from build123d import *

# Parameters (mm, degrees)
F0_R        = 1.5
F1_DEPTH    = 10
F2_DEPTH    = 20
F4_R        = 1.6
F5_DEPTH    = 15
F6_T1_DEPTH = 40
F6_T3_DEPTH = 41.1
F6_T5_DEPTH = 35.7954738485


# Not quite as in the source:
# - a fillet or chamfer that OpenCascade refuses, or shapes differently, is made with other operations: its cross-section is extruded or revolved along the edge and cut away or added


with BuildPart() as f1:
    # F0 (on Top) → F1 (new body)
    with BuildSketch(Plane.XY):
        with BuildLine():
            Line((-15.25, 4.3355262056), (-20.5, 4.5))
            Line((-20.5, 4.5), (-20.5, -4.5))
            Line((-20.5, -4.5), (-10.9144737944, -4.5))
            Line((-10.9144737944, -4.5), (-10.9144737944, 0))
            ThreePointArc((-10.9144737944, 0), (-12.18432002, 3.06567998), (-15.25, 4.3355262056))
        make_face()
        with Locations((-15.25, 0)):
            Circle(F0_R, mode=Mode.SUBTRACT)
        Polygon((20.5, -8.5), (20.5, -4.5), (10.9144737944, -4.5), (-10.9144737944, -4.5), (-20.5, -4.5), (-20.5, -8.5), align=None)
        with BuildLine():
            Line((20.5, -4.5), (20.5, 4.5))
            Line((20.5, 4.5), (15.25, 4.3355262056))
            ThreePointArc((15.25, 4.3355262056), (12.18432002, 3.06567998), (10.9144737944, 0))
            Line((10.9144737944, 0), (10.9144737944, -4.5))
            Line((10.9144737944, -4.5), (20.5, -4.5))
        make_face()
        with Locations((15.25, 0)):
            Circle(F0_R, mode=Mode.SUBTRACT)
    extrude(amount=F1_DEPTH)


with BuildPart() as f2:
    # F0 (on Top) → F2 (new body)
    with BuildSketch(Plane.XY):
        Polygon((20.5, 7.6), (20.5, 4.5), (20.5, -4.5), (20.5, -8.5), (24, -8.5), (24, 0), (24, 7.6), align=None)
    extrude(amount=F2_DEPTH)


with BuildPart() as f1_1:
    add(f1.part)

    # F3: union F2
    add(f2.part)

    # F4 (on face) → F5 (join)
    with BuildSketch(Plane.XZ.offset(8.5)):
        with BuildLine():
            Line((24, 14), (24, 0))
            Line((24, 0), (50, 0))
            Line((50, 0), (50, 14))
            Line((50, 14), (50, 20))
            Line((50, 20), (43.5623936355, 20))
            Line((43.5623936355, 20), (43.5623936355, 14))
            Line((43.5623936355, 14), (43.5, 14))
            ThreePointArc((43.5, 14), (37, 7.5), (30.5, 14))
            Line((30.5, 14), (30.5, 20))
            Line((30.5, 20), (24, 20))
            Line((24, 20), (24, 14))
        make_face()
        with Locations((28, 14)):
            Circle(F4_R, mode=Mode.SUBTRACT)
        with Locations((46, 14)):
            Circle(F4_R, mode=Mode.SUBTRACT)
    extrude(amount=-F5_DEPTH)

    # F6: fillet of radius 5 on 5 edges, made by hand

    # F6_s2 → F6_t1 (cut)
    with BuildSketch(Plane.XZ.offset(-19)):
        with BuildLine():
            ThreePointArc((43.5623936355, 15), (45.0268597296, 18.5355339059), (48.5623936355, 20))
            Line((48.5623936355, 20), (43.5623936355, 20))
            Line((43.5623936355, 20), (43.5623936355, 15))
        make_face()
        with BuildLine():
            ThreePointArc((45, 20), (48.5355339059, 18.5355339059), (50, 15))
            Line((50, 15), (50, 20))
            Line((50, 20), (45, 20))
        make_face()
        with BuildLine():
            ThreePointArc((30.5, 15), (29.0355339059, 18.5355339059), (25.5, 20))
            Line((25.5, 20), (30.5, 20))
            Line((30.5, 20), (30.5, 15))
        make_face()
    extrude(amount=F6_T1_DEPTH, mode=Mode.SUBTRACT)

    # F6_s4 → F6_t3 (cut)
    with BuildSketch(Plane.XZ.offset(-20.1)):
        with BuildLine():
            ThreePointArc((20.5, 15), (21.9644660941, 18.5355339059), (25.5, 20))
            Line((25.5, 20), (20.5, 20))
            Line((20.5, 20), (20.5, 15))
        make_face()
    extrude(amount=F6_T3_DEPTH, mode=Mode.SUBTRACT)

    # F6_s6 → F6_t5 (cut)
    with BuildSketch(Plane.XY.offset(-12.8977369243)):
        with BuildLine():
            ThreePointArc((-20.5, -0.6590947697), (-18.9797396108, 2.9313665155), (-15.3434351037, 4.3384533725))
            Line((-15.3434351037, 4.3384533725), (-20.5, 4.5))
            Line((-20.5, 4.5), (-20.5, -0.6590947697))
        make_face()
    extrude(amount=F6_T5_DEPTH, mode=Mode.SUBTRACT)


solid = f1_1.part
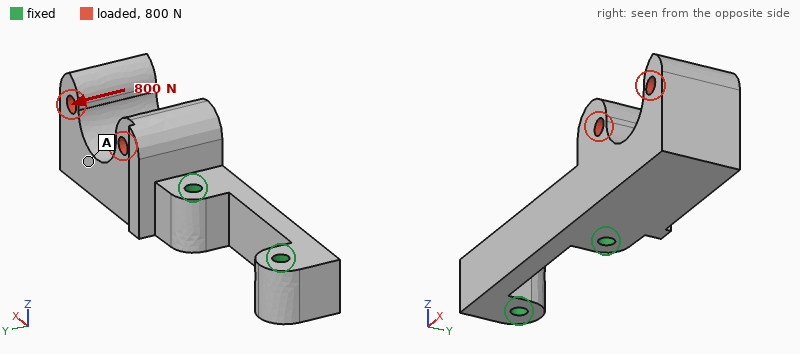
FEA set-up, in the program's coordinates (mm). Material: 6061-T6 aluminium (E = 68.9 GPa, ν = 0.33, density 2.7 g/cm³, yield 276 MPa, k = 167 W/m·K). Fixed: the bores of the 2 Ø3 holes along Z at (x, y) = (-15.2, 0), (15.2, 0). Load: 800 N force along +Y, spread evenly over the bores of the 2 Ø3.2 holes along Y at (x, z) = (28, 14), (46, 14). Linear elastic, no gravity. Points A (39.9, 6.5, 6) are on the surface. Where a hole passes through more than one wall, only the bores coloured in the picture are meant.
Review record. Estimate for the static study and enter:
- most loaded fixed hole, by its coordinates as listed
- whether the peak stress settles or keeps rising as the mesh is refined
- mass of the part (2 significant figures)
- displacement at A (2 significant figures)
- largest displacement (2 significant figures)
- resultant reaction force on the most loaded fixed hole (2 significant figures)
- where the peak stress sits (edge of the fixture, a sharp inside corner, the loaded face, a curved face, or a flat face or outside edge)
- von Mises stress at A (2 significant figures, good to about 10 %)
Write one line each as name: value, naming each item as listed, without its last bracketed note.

most loaded fixed hole, by its coordinates as listed: (15.2, 0)
whether the peak stress settles or keeps rising as the mesh is refined: keeps rising
mass of the part: 25 g
displacement at A: 0.070 mm
largest displacement: 0.12 mm
resultant reaction force on the most loaded fixed hole: 1.1 kN
where the peak stress sits: edge of the fixture
von Mises stress at A: 23 MPa
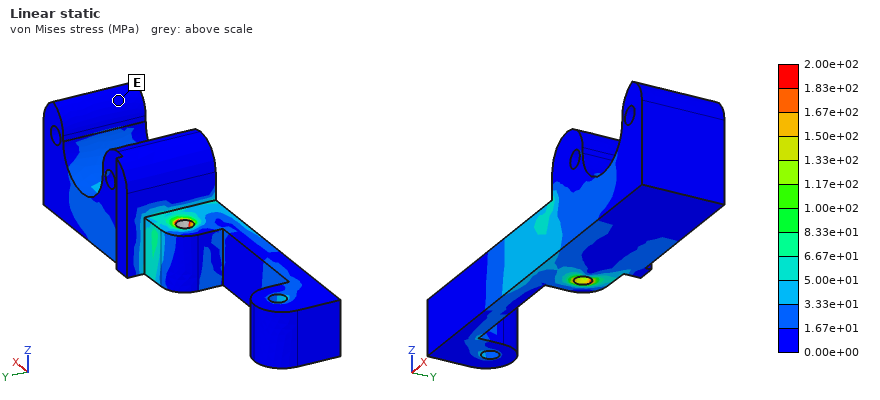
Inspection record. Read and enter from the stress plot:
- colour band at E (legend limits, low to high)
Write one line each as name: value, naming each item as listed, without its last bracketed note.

colour band at E: 0.00e+00 to 1.67e+01 MPa
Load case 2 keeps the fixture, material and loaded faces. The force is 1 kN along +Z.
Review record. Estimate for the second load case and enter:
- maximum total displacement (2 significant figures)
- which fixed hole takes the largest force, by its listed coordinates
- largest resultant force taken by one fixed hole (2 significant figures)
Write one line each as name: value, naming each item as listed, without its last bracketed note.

maximum total displacement: 0.12 mm
which fixed hole takes the largest force, by its listed coordinates: (15.2, 0)
largest resultant force taken by one fixed hole: 1.1 kN
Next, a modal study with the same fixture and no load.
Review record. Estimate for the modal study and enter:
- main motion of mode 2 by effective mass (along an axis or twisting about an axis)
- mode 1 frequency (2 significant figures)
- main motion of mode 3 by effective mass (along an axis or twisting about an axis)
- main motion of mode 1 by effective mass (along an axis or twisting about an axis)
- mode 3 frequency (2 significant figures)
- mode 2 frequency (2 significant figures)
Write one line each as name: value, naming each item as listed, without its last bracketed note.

main motion of mode 2 by effective mass: along Z
mode 1 frequency: 4500 Hz
main motion of mode 3 by effective mass: twisting about X
main motion of mode 1 by effective mass: along Y
mode 3 frequency: 12 kHz
mode 2 frequency: 4800 Hz
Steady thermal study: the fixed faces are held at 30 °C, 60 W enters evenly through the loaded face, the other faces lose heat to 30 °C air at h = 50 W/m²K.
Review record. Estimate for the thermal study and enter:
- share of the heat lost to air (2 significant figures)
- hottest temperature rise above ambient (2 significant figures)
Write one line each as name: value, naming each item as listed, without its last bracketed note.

share of the heat lost to air: 8.2 %
hottest temperature rise above ambient: 64 K
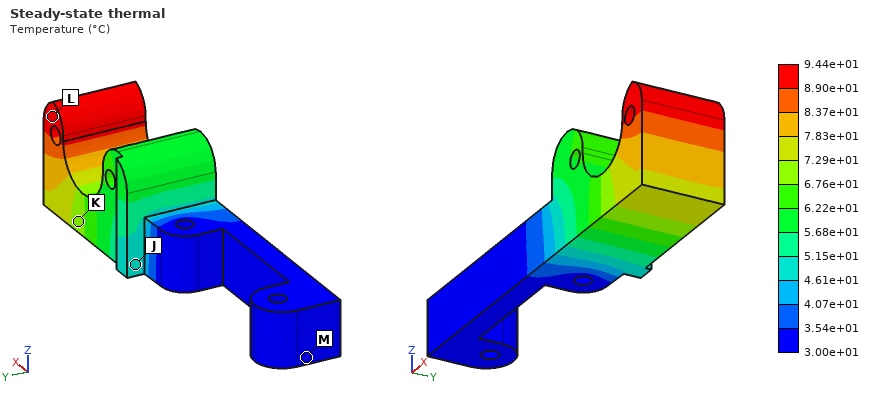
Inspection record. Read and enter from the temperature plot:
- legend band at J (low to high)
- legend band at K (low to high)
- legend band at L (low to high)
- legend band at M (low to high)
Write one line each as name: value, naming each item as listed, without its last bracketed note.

legend band at J: 4.61e+01 to 5.15e+01 °C
legend band at K: 6.76e+01 to 7.29e+01 °C
legend band at L: 8.90e+01 to 9.44e+01 °C
legend band at M: 3.00e+01 to 3.54e+01 °C
